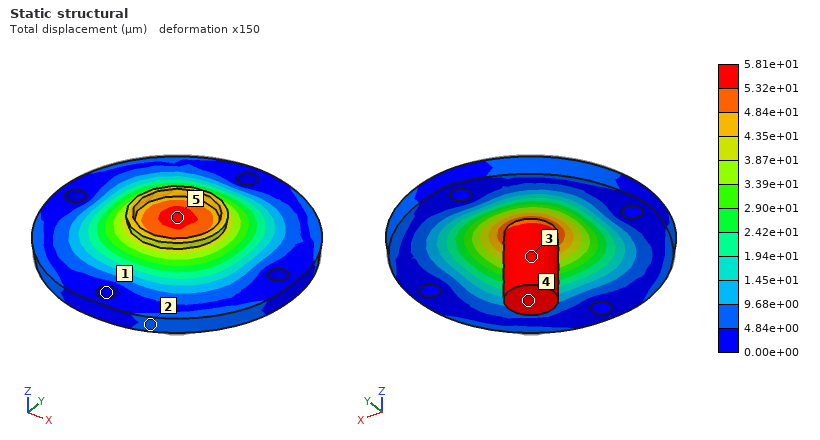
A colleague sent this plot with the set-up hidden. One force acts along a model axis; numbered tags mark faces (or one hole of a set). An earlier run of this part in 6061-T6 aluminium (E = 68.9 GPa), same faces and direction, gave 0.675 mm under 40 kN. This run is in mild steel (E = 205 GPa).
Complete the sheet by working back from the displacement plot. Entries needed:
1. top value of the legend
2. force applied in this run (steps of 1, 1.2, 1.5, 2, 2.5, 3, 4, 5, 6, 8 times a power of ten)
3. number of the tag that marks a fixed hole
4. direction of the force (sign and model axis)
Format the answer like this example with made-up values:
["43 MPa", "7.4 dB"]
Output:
["5.81e+01 µm", "10 kN", "1", "+Z"]
